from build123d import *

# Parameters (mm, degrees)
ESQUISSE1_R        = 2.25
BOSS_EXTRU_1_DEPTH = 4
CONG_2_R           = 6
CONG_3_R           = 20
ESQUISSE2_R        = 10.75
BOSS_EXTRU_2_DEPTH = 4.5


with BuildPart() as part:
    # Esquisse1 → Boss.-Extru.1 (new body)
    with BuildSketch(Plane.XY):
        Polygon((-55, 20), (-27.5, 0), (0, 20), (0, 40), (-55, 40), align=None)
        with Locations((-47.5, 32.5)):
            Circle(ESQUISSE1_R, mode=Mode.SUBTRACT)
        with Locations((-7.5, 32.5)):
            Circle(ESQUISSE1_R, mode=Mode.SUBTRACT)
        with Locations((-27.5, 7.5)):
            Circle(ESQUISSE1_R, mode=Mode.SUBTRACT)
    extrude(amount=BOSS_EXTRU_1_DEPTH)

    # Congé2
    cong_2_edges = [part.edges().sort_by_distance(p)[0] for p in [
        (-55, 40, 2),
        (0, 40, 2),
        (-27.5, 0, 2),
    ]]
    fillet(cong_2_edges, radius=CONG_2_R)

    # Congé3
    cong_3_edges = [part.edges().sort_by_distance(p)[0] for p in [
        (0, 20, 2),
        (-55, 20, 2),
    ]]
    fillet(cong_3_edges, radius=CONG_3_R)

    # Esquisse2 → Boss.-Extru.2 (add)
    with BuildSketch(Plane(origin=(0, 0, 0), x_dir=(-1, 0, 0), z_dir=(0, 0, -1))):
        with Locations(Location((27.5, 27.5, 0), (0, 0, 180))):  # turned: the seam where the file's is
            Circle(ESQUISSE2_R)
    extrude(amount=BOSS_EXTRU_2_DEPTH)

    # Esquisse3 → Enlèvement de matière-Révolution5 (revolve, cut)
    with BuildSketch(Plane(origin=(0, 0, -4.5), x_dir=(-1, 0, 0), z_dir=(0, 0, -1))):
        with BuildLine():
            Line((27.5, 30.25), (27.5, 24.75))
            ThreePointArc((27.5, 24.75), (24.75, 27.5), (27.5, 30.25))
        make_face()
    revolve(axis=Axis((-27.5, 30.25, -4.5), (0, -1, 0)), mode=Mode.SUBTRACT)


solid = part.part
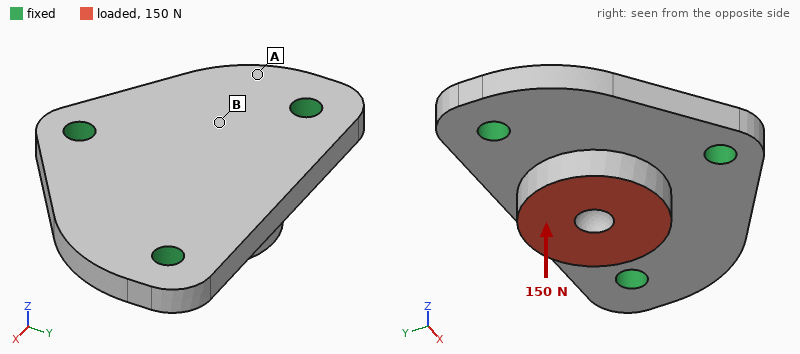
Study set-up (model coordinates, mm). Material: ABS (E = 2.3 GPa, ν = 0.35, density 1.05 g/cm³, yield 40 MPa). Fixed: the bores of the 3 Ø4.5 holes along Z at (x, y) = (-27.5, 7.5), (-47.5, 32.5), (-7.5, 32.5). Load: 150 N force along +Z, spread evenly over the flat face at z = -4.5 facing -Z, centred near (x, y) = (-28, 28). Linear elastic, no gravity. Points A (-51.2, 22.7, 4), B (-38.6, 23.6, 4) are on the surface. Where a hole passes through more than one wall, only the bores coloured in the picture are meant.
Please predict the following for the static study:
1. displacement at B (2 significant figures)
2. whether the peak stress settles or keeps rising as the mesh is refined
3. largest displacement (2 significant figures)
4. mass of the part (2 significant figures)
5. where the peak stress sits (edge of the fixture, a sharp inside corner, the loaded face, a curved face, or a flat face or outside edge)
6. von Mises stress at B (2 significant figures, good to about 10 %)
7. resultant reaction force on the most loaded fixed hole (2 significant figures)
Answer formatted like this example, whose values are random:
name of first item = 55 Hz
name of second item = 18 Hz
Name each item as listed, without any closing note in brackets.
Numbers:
displacement at B = 33 µm
whether the peak stress settles or keeps rising as the mesh is refined = keeps rising
largest displacement = 78 µm
mass of the part = 8.2 g
where the peak stress sits = edge of the fixture
von Mises stress at B = 2.0 MPa
resultant reaction force on the most loaded fixed hole = 62 N
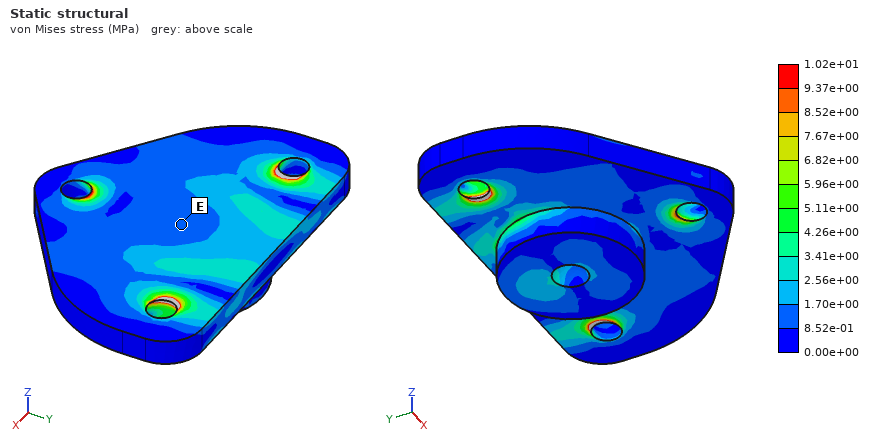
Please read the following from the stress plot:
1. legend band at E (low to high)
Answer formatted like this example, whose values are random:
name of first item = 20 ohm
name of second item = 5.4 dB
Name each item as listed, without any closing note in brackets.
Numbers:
legend band at E = 8.52e-01 to 1.70e+00 MPa
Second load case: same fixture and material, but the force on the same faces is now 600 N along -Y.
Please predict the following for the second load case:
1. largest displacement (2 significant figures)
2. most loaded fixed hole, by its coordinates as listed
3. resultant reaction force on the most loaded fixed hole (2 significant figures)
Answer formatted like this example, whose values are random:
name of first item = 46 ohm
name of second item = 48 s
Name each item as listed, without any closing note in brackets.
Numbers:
largest displacement = 0.24 mm
most loaded fixed hole, by its coordinates as listed = (-27.5, 7.5)
resultant reaction force on the most loaded fixed hole = 360 N
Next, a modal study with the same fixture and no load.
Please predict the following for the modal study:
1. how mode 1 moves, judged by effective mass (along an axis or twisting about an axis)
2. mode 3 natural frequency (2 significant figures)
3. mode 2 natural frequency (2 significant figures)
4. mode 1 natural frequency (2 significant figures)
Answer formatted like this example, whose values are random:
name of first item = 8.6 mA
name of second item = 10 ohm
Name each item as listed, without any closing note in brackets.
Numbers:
how mode 1 moves, judged by effective mass = along Z
mode 3 natural frequency = 5400 Hz
mode 2 natural frequency = 5300 Hz
mode 1 natural frequency = 4100 Hz
